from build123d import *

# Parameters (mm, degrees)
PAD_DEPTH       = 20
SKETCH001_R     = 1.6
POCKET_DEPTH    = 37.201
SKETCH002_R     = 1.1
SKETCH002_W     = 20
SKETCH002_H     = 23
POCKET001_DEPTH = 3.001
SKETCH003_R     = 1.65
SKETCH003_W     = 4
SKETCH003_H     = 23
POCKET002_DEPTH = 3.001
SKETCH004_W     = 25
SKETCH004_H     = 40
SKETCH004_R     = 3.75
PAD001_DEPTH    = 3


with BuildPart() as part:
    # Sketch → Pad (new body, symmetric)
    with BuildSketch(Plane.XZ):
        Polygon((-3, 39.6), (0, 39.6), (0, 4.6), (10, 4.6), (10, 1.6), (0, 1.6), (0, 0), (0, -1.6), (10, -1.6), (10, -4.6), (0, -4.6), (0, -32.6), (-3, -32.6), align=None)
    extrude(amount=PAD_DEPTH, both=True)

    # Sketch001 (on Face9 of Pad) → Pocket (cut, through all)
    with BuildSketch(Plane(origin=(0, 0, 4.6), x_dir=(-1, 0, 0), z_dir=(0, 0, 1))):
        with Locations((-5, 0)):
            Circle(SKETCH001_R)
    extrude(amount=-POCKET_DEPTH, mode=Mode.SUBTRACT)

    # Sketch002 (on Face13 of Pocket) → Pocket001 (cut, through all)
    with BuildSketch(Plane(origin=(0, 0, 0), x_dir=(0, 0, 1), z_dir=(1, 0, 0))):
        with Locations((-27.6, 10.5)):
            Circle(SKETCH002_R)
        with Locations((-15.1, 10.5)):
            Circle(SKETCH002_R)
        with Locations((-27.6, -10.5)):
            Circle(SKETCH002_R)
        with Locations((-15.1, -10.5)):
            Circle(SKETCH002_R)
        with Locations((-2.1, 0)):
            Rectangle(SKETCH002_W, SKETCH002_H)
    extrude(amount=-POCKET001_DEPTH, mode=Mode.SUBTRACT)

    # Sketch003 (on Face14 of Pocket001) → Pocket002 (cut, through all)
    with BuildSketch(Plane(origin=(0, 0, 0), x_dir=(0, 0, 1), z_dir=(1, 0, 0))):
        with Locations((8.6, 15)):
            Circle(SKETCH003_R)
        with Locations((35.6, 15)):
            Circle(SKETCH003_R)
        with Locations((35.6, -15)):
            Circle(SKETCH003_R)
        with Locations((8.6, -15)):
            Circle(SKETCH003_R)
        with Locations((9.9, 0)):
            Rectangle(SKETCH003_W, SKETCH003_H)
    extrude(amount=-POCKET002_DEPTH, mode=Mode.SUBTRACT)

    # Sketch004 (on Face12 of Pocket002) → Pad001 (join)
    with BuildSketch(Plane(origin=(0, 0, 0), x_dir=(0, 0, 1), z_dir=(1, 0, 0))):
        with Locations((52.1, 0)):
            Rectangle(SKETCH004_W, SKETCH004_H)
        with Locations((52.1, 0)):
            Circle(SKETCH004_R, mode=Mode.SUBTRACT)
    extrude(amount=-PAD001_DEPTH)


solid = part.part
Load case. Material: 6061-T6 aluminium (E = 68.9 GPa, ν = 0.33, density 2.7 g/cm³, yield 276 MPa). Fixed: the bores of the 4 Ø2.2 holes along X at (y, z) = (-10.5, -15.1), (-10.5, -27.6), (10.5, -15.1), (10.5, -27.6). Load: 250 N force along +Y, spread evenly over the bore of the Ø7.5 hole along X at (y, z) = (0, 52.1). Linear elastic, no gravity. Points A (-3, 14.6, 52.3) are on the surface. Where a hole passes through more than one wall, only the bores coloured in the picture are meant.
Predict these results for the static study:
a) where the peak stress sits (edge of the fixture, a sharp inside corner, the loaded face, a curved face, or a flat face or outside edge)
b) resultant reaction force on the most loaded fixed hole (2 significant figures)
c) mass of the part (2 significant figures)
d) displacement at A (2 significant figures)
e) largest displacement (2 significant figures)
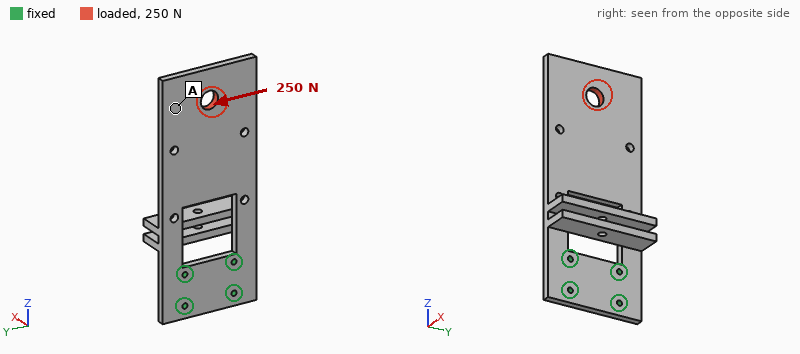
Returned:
a curved face
410 N
33 g
86 µm
99 µm
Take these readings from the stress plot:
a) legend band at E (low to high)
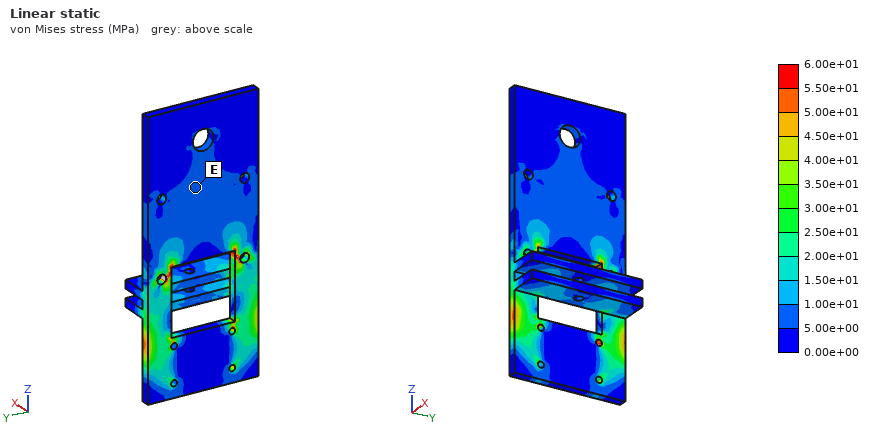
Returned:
5.00e+00 to 1.00e+01 MPa
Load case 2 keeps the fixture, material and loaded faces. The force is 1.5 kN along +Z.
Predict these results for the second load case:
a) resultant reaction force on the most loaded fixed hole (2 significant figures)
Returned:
540 N
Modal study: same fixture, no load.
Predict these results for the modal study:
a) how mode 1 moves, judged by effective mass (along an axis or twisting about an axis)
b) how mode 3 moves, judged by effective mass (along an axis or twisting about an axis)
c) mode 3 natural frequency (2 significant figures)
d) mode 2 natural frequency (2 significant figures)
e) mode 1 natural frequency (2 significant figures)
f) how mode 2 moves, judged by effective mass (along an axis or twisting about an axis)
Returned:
along X
along X
1800 Hz
1500 Hz
260 Hz
twisting about Z
